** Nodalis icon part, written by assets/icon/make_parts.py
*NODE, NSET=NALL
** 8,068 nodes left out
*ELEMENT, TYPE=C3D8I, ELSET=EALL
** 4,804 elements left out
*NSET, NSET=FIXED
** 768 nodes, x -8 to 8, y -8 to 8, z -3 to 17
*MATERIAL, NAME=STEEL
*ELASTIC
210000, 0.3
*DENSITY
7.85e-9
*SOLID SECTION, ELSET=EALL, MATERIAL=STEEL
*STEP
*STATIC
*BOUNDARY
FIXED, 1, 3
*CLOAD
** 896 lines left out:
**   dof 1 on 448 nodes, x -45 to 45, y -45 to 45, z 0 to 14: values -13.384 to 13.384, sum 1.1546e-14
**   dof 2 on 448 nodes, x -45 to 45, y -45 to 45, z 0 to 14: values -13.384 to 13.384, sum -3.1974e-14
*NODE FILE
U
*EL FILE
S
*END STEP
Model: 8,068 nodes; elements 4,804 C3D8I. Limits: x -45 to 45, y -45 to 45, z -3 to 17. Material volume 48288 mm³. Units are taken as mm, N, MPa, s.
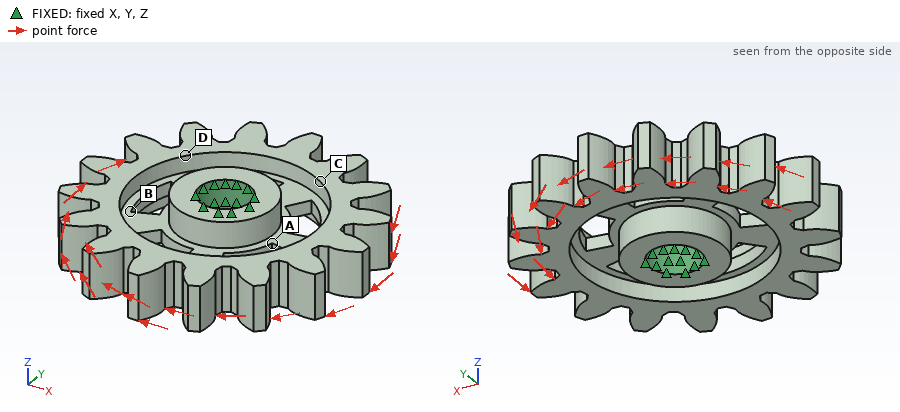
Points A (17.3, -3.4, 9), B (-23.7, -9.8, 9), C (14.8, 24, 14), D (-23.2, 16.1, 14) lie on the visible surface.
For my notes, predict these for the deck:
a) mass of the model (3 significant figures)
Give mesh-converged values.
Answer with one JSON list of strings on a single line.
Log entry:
["0.379 kg"]
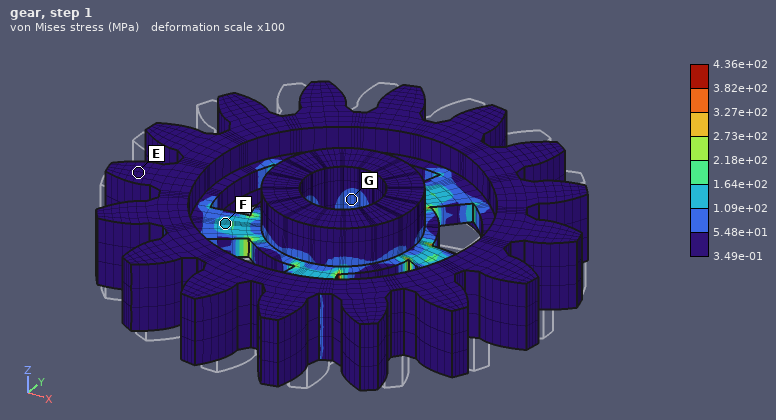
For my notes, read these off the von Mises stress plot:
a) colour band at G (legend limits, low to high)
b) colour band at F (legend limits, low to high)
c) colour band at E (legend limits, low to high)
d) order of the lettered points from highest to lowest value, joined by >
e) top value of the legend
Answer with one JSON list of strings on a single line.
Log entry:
["5.48e+01 to 1.09e+02 MPa", "1.09e+02 to 1.64e+02 MPa", "3.49e-01 to 5.48e+01 MPa", "F > G > E", "4.36e+02 MPa"]
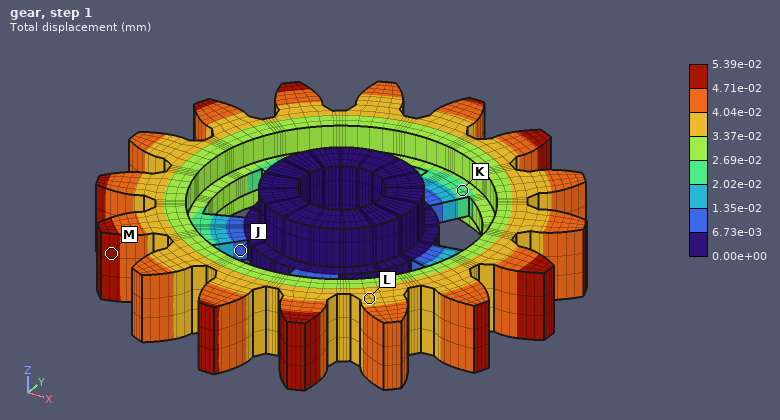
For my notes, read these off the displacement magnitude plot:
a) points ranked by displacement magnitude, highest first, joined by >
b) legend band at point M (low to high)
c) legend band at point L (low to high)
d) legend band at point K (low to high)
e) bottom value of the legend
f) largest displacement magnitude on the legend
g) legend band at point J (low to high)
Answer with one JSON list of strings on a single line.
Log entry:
["M > L > K > J", "4.71e-02 to 5.39e-02 mm", "3.37e-02 to 4.04e-02 mm", "2.02e-02 to 2.69e-02 mm", "0.00e+00 mm", "5.39e-02 mm", "6.73e-03 to 1.35e-02 mm"]
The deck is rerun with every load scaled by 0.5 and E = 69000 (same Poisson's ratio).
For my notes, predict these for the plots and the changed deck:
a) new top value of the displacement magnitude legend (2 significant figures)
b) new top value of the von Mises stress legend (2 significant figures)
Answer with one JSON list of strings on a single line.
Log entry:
["0.082 mm", "220 MPa"]
